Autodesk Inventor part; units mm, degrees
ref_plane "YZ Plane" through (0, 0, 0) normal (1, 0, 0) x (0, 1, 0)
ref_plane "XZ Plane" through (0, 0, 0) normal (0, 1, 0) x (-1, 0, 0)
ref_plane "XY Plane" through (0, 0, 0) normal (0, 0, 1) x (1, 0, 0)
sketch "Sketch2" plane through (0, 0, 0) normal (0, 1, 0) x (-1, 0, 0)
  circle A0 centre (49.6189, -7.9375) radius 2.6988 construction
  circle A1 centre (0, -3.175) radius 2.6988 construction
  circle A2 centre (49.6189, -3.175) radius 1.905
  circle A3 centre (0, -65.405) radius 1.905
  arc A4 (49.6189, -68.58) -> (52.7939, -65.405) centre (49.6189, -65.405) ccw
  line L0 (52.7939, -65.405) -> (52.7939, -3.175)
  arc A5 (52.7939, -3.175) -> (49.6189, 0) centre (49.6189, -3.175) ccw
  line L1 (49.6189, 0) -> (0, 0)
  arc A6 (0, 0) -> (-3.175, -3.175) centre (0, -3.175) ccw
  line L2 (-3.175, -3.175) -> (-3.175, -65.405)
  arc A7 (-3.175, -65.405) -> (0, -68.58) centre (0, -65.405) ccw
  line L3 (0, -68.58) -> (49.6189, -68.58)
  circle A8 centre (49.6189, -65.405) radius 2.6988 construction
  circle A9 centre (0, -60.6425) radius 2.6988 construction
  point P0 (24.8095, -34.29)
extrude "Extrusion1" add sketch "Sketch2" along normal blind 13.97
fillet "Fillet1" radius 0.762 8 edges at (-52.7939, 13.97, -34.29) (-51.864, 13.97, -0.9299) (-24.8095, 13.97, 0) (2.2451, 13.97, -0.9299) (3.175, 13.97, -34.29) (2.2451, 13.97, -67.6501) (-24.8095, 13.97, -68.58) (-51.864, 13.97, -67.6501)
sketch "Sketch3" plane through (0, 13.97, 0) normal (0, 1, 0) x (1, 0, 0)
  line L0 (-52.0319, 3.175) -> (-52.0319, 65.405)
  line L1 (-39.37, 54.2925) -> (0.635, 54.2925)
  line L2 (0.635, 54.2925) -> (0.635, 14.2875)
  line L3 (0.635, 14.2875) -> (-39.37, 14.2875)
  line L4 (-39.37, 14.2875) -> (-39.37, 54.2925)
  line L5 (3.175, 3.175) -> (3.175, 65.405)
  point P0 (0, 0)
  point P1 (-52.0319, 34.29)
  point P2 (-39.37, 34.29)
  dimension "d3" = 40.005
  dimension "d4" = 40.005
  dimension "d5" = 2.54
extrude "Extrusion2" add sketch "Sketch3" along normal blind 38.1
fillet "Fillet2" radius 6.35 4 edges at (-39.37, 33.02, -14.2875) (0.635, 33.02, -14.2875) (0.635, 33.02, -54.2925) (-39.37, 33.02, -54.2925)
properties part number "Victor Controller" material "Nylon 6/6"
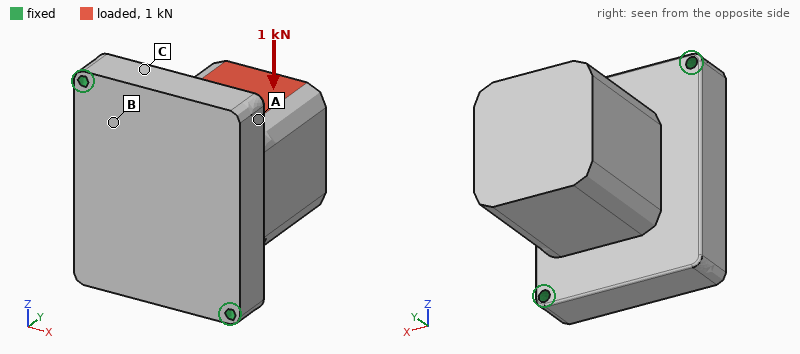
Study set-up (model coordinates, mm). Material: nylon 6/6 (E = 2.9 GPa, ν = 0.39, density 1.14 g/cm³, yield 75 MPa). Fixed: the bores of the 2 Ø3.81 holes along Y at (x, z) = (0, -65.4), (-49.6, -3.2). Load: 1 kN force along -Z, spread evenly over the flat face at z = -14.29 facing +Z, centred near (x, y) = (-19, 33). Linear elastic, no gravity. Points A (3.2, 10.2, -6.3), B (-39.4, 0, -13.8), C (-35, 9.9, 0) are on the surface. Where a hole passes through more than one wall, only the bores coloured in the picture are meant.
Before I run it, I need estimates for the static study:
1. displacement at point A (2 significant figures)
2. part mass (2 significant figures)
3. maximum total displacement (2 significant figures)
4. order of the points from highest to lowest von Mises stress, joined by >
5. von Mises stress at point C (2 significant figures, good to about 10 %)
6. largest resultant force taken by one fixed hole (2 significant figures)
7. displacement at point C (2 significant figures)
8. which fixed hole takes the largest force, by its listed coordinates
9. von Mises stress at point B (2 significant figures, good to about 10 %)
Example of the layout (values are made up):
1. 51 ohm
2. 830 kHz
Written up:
1. 0.57 mm
2. 130 g
3. 0.80 mm
4. C > B > A
5. 9.0 MPa
6. 630 N
7. 0.16 mm
8. (0, -65.4)
9. 5.0 MPa
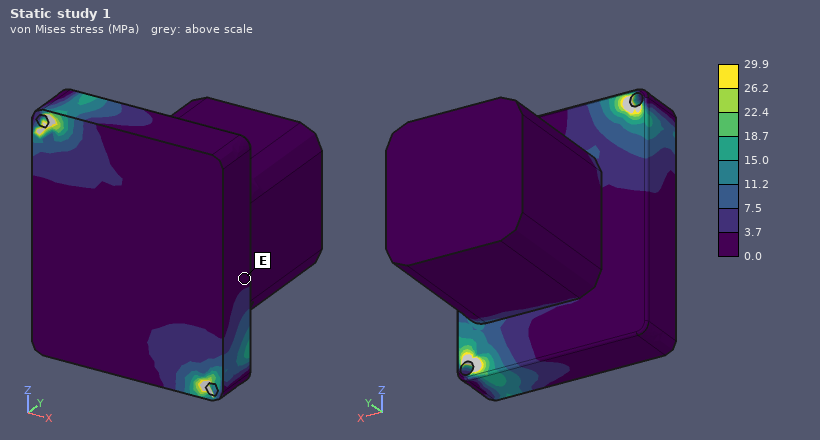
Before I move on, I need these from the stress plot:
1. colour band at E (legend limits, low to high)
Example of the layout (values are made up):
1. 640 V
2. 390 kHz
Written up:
1. 0.0 to 3.7 MPa
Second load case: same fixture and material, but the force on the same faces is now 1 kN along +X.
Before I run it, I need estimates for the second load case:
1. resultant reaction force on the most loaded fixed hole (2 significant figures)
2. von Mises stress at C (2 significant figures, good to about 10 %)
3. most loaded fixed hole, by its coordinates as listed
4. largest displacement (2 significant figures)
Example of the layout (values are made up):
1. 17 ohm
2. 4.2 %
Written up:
1. 760 N
2. 11 MPa
3. (-49.6, -3.2)
4. 1.0 mm
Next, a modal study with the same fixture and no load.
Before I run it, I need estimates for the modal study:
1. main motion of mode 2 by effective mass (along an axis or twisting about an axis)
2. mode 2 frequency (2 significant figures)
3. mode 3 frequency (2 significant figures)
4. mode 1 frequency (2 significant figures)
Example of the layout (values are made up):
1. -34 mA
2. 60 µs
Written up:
1. along Y
2. 1500 Hz
3. 2000 Hz
4. 580 Hz
